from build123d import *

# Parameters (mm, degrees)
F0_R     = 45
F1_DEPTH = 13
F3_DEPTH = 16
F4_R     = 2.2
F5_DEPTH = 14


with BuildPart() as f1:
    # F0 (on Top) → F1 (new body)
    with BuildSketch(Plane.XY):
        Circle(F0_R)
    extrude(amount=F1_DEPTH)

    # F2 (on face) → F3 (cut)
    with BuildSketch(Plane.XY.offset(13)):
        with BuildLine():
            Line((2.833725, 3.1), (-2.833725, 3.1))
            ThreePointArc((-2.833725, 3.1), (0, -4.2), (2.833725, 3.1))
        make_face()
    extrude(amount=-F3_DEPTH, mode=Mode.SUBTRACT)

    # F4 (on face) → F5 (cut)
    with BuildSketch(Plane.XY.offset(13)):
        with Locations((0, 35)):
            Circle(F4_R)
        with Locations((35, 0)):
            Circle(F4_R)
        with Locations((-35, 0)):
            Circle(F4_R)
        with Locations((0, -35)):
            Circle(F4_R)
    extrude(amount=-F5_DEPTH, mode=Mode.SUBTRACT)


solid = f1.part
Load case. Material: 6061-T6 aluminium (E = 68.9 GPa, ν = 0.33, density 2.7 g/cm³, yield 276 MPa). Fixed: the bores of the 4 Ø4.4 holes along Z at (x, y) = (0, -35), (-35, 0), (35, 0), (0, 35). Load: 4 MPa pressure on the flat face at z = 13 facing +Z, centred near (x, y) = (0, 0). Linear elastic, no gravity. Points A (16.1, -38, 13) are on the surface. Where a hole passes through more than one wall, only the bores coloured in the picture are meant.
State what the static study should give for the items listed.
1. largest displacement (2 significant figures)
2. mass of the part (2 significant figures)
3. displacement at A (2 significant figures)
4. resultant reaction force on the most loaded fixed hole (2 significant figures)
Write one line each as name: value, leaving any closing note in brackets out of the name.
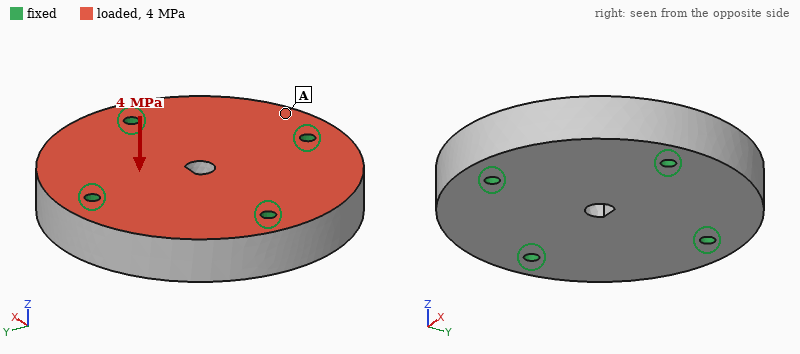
largest displacement: 21 µm
mass of the part: 220 g
displacement at A: 11 µm
resultant reaction force on the most loaded fixed hole: 6.3 kN
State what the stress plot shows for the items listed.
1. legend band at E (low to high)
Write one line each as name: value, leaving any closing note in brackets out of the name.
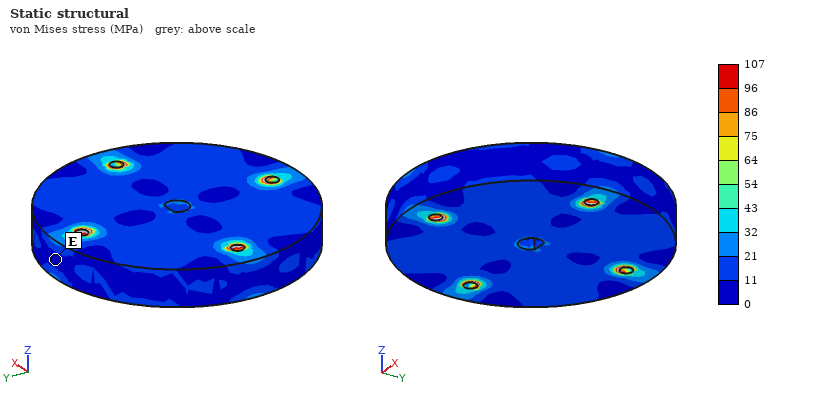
legend band at E: 0 to 11 MPa
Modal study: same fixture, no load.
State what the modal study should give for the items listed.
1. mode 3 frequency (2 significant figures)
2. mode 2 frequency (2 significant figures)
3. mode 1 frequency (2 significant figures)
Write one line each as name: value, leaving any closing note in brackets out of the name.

mode 3 frequency: 15 kHz
mode 2 frequency: 14 kHz
mode 1 frequency: 13 kHz
